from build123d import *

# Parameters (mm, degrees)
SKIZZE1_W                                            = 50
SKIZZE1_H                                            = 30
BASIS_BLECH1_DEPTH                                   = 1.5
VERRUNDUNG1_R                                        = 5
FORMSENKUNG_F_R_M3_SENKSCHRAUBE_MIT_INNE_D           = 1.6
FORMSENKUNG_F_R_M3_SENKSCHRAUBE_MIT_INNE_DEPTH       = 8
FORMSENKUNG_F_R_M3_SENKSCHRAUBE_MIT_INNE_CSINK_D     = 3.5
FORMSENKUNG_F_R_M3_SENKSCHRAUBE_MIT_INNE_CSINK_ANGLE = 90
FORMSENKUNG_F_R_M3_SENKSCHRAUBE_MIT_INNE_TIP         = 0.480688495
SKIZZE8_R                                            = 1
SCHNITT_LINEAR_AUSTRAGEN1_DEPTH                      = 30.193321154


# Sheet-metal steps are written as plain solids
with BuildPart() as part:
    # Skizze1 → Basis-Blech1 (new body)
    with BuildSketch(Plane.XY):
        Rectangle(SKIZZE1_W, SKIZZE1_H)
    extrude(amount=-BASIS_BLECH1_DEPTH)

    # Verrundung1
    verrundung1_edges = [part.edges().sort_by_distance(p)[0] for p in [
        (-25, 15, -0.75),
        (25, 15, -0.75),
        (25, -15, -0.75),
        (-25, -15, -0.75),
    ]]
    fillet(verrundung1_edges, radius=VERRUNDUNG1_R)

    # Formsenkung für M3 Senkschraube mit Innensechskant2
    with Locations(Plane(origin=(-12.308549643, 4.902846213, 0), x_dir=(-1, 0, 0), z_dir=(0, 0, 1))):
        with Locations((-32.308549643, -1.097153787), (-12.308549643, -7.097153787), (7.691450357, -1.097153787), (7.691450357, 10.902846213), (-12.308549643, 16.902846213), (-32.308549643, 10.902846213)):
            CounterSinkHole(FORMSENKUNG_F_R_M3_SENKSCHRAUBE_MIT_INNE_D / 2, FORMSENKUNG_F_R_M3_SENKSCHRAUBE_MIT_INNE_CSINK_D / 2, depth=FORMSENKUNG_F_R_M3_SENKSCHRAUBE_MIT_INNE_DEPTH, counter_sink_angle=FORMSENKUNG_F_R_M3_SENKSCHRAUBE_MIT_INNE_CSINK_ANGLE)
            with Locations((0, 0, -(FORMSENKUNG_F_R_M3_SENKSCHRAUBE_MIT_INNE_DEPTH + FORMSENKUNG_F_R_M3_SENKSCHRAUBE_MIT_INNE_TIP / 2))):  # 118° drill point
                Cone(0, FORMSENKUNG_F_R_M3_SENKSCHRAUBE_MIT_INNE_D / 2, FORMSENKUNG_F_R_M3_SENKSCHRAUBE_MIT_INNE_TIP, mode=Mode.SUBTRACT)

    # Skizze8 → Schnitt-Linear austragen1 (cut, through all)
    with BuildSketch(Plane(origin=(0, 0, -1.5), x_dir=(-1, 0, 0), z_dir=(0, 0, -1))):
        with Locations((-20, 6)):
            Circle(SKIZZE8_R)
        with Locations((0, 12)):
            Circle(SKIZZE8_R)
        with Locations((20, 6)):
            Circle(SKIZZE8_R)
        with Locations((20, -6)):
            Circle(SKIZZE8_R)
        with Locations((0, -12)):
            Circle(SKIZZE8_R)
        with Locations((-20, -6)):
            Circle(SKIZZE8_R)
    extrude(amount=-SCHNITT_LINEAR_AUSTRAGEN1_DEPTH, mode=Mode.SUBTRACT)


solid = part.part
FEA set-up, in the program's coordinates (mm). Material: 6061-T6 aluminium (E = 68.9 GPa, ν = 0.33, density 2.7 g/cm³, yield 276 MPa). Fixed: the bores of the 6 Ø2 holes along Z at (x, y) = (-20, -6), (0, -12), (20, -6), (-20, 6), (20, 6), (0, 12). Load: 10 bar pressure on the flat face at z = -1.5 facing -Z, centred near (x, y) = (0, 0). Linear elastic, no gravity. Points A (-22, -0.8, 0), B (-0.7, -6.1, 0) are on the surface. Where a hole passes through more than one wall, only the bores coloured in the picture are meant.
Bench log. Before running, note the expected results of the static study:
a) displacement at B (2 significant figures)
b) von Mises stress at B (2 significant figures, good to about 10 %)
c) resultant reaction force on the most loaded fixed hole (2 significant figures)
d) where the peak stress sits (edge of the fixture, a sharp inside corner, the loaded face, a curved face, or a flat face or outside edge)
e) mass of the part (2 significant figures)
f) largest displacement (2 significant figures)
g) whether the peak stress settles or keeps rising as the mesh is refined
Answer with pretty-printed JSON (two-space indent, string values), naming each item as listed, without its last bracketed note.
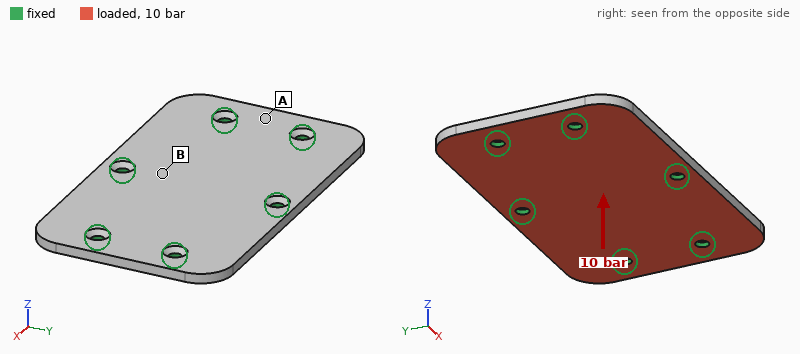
{
  "displacement at B": "40 µm",
  "von Mises stress at B": "58 MPa",
  "resultant reaction force on the most loaded fixed hole": "330 N",
  "where the peak stress sits": "edge of the fixture",
  "mass of the part": "5.9 g",
  "largest displacement": "63 µm",
  "whether the peak stress settles or keeps rising as the mesh is refined": "keeps rising"
}
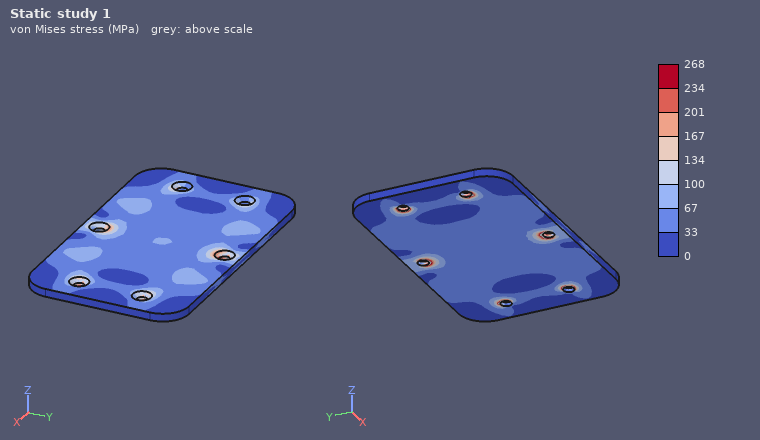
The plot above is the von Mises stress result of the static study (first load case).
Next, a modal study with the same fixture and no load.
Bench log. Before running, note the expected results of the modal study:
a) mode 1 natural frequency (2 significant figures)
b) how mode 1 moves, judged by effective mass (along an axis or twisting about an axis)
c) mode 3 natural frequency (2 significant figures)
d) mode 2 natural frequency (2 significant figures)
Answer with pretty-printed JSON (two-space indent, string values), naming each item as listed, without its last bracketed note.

{
  "mode 1 natural frequency": "11 kHz",
  "how mode 1 moves, judged by effective mass": "along Z",
  "mode 3 natural frequency": "13 kHz",
  "mode 2 natural frequency": "12 kHz"
}
